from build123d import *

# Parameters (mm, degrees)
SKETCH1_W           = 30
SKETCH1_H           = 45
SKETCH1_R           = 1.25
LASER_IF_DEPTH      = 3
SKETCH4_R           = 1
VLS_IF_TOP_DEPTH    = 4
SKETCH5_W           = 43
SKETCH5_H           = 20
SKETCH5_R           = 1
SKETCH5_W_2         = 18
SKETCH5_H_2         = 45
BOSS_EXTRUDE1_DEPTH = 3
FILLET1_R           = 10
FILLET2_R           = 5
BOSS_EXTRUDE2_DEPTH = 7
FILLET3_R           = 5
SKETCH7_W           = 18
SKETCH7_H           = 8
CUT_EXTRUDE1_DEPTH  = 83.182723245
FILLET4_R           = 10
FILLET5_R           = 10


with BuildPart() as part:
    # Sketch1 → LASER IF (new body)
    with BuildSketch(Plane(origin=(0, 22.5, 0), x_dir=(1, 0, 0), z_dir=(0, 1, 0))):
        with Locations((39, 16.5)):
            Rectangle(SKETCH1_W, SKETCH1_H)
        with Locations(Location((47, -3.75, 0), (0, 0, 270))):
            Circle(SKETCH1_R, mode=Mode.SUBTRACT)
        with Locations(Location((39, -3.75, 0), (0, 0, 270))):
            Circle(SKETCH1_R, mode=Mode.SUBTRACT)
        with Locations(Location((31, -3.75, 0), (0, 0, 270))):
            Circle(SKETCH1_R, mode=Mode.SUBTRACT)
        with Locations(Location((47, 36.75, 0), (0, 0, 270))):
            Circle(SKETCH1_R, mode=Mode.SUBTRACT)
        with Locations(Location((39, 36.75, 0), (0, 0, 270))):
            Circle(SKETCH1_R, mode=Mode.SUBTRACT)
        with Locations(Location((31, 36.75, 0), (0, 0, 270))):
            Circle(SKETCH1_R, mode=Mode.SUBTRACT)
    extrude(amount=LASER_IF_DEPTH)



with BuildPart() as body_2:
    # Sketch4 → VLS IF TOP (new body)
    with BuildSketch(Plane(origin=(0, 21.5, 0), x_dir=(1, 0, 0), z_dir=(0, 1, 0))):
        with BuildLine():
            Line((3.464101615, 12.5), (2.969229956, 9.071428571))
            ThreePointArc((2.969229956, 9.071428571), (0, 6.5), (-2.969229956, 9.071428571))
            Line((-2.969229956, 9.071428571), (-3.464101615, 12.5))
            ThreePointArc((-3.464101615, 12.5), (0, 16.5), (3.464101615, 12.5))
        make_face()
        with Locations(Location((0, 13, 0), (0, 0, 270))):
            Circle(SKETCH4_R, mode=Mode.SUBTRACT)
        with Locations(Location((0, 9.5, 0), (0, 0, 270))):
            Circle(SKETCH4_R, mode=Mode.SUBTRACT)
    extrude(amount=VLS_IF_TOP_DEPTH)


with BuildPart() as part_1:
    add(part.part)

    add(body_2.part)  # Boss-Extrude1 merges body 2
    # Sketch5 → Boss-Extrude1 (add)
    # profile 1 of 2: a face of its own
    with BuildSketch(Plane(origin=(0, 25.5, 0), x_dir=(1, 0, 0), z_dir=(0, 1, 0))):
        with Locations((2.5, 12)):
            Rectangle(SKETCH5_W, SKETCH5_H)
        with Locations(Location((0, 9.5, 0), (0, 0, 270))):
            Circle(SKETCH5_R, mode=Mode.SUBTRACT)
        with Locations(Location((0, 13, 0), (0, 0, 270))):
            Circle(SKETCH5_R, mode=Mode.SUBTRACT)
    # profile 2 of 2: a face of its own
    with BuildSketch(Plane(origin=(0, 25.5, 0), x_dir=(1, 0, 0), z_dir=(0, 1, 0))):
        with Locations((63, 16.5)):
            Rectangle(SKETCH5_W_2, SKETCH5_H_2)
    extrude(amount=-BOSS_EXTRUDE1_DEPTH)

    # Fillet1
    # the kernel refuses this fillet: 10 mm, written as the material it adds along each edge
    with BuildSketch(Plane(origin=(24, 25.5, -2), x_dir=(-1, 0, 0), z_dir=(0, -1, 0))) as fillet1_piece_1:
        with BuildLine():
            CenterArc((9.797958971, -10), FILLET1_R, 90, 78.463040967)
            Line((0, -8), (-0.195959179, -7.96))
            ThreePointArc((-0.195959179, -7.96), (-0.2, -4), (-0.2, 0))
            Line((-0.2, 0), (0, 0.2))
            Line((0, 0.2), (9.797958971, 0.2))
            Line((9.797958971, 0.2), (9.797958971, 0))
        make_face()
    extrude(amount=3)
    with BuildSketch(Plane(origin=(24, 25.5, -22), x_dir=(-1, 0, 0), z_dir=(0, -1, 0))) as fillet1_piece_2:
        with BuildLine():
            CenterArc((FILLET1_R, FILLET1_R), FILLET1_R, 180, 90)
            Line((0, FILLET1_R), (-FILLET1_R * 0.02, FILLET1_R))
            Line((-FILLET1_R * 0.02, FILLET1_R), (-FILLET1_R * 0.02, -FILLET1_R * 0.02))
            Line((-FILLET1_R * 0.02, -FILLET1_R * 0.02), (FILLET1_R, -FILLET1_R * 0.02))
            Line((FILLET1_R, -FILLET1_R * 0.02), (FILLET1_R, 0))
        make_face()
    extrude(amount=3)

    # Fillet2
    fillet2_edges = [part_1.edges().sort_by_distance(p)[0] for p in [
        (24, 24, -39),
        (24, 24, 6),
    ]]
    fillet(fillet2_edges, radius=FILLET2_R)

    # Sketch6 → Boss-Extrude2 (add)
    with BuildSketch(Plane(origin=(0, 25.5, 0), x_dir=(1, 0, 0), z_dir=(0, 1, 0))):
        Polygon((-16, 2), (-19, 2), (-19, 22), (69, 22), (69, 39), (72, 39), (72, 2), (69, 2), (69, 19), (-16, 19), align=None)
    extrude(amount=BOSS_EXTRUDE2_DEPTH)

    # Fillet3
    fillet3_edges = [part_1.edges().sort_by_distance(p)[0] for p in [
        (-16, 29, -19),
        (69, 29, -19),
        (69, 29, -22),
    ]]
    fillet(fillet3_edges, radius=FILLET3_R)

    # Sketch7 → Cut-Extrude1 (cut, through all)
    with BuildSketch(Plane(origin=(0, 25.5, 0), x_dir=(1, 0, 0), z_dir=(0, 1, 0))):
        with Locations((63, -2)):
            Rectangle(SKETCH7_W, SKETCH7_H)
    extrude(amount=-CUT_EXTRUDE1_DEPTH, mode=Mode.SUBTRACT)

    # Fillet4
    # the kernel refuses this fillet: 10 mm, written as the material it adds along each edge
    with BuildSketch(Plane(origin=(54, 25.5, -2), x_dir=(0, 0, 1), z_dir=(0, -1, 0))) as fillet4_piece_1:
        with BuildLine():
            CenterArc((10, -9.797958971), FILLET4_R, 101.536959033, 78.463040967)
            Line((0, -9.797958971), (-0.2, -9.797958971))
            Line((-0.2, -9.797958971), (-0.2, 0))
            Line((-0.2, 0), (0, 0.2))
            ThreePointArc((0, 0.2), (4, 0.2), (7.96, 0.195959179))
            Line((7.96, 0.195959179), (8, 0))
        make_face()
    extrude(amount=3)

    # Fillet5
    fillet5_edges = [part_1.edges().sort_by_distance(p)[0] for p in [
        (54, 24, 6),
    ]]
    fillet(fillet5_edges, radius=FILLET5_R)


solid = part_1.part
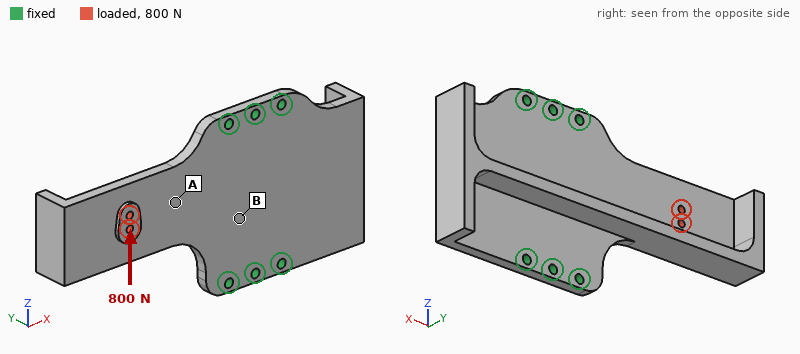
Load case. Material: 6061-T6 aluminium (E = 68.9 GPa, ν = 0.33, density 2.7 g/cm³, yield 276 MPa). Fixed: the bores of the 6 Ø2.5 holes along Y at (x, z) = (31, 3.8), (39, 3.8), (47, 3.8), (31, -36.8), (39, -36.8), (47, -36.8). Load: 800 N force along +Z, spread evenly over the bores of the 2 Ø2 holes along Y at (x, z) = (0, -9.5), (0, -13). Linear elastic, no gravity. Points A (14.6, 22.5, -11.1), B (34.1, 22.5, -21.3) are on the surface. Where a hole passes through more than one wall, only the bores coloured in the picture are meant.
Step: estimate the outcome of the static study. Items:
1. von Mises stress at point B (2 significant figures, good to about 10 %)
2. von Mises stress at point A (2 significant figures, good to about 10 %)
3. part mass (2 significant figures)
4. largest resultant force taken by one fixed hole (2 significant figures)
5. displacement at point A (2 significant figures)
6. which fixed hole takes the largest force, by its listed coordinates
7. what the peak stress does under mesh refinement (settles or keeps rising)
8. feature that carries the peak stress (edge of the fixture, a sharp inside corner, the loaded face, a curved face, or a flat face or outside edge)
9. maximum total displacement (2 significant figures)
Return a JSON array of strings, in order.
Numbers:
["13 MPa", "32 MPa", "32 g", "710 N", "0.018 mm", "(31, 3.8)", "keeps rising", "edge of the fixture", "0.11 mm"]
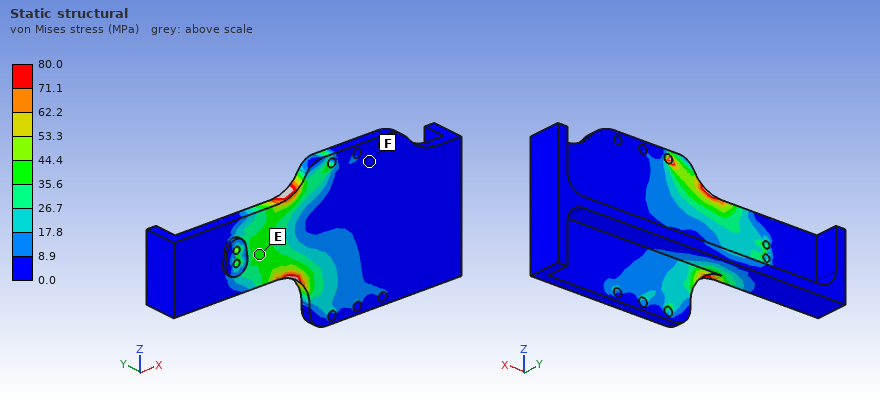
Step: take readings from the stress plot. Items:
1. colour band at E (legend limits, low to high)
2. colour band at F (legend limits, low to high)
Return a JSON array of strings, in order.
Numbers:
["35.6 to 44.4 MPa", "0.0 to 8.9 MPa"]
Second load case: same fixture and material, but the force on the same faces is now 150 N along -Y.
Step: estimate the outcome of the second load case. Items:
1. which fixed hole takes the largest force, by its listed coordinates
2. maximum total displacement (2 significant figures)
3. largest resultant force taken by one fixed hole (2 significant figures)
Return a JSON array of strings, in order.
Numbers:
["(31, 3.8)", "0.30 mm", "190 N"]
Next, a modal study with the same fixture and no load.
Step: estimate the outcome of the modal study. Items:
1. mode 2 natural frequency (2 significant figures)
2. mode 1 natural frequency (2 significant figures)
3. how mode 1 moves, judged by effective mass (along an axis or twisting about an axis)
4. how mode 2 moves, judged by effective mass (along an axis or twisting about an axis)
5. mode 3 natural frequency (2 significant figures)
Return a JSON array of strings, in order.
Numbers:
["3200 Hz", "1400 Hz", "along Y", "along Y", "4000 Hz"]
